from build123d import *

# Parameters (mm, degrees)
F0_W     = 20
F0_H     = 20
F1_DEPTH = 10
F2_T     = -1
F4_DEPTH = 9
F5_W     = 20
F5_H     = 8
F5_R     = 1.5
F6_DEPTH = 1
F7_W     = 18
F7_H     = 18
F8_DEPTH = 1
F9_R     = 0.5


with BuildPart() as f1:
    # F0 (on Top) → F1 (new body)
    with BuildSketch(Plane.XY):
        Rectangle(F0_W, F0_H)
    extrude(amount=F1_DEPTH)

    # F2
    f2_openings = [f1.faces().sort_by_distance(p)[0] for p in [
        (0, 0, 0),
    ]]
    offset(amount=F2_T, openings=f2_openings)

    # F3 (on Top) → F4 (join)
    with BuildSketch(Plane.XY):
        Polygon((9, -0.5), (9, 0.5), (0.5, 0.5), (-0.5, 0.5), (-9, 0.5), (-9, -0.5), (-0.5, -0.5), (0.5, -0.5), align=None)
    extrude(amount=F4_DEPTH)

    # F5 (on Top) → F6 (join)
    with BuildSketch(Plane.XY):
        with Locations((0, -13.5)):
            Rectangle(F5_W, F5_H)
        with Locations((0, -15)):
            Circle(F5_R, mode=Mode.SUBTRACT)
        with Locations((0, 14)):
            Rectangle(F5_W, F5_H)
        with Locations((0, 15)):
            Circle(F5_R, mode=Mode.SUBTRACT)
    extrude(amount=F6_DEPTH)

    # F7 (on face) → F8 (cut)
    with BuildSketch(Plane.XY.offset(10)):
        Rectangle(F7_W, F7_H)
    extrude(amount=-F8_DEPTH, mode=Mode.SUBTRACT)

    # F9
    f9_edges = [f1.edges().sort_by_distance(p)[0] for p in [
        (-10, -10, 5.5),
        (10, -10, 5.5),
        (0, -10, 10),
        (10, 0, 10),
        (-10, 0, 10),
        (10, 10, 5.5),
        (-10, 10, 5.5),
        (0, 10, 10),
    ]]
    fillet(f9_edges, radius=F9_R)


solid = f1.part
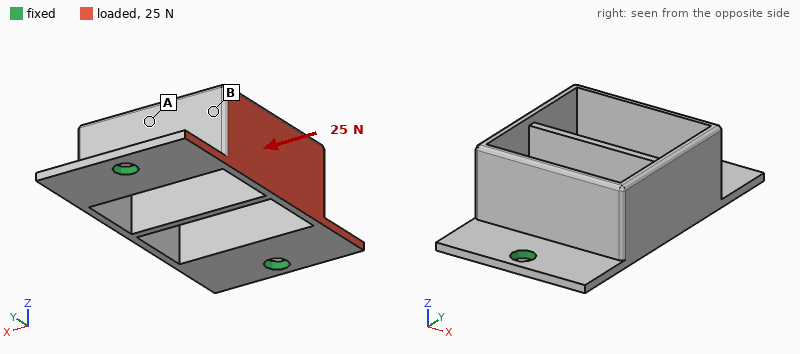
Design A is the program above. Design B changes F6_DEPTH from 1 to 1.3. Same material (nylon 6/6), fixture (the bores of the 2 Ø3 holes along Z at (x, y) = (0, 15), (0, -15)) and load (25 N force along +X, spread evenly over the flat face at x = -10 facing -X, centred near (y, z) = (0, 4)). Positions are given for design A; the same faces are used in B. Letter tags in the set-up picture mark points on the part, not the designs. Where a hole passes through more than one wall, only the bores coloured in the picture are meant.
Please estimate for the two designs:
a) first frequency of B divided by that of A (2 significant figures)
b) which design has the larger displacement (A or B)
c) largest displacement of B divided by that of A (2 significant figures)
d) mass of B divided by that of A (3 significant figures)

1.3
A
0.63
1.07
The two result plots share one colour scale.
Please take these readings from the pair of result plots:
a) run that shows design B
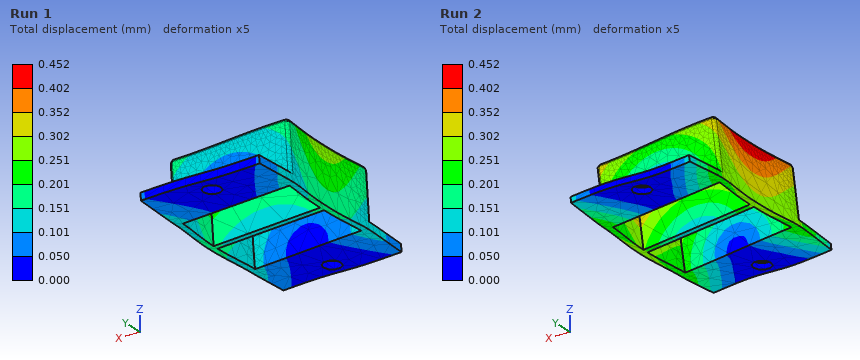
Run 1
